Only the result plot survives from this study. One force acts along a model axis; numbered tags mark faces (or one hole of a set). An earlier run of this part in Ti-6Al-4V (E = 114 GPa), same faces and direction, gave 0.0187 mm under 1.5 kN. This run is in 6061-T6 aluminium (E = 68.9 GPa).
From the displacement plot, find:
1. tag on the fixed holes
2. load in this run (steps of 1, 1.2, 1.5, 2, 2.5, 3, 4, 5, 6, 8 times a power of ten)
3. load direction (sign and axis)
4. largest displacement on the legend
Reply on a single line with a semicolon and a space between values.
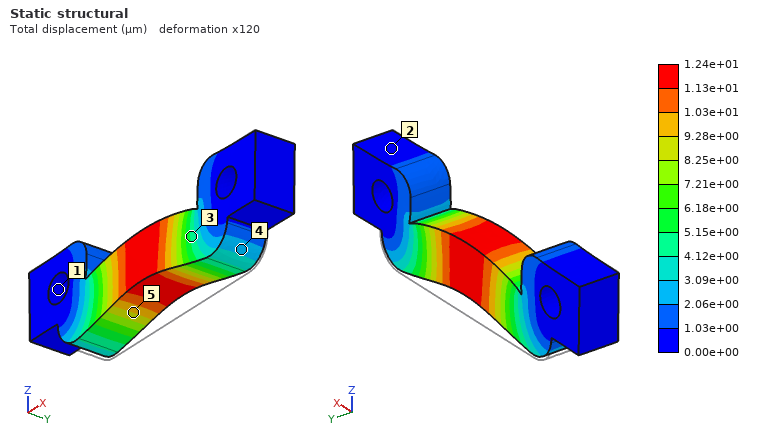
1; 600 N; +Z; 1.24e+01 µm
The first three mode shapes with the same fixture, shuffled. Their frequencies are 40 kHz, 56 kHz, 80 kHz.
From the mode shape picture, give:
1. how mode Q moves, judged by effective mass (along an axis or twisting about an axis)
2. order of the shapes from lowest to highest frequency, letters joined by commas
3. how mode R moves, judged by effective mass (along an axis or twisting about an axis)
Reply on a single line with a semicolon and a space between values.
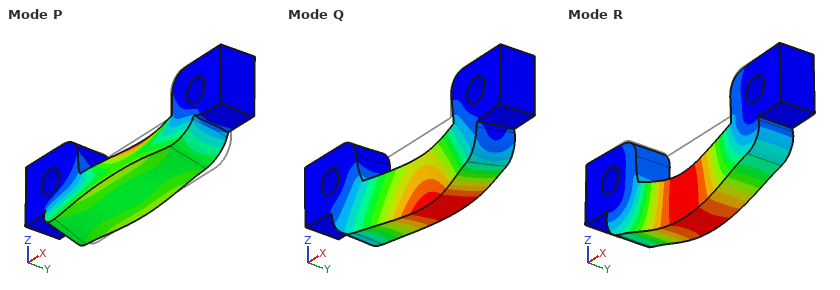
along Y; Q, R, P; along Z
